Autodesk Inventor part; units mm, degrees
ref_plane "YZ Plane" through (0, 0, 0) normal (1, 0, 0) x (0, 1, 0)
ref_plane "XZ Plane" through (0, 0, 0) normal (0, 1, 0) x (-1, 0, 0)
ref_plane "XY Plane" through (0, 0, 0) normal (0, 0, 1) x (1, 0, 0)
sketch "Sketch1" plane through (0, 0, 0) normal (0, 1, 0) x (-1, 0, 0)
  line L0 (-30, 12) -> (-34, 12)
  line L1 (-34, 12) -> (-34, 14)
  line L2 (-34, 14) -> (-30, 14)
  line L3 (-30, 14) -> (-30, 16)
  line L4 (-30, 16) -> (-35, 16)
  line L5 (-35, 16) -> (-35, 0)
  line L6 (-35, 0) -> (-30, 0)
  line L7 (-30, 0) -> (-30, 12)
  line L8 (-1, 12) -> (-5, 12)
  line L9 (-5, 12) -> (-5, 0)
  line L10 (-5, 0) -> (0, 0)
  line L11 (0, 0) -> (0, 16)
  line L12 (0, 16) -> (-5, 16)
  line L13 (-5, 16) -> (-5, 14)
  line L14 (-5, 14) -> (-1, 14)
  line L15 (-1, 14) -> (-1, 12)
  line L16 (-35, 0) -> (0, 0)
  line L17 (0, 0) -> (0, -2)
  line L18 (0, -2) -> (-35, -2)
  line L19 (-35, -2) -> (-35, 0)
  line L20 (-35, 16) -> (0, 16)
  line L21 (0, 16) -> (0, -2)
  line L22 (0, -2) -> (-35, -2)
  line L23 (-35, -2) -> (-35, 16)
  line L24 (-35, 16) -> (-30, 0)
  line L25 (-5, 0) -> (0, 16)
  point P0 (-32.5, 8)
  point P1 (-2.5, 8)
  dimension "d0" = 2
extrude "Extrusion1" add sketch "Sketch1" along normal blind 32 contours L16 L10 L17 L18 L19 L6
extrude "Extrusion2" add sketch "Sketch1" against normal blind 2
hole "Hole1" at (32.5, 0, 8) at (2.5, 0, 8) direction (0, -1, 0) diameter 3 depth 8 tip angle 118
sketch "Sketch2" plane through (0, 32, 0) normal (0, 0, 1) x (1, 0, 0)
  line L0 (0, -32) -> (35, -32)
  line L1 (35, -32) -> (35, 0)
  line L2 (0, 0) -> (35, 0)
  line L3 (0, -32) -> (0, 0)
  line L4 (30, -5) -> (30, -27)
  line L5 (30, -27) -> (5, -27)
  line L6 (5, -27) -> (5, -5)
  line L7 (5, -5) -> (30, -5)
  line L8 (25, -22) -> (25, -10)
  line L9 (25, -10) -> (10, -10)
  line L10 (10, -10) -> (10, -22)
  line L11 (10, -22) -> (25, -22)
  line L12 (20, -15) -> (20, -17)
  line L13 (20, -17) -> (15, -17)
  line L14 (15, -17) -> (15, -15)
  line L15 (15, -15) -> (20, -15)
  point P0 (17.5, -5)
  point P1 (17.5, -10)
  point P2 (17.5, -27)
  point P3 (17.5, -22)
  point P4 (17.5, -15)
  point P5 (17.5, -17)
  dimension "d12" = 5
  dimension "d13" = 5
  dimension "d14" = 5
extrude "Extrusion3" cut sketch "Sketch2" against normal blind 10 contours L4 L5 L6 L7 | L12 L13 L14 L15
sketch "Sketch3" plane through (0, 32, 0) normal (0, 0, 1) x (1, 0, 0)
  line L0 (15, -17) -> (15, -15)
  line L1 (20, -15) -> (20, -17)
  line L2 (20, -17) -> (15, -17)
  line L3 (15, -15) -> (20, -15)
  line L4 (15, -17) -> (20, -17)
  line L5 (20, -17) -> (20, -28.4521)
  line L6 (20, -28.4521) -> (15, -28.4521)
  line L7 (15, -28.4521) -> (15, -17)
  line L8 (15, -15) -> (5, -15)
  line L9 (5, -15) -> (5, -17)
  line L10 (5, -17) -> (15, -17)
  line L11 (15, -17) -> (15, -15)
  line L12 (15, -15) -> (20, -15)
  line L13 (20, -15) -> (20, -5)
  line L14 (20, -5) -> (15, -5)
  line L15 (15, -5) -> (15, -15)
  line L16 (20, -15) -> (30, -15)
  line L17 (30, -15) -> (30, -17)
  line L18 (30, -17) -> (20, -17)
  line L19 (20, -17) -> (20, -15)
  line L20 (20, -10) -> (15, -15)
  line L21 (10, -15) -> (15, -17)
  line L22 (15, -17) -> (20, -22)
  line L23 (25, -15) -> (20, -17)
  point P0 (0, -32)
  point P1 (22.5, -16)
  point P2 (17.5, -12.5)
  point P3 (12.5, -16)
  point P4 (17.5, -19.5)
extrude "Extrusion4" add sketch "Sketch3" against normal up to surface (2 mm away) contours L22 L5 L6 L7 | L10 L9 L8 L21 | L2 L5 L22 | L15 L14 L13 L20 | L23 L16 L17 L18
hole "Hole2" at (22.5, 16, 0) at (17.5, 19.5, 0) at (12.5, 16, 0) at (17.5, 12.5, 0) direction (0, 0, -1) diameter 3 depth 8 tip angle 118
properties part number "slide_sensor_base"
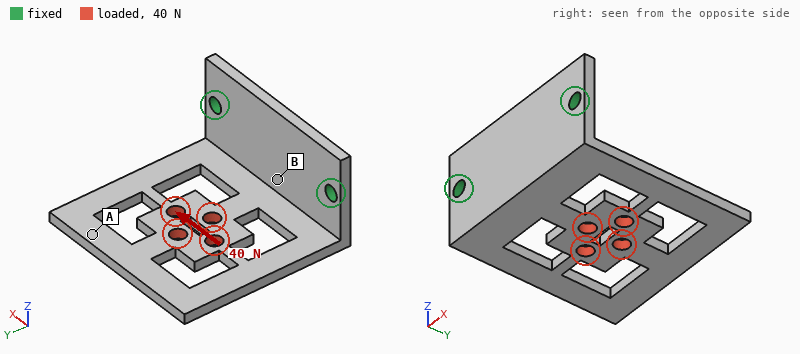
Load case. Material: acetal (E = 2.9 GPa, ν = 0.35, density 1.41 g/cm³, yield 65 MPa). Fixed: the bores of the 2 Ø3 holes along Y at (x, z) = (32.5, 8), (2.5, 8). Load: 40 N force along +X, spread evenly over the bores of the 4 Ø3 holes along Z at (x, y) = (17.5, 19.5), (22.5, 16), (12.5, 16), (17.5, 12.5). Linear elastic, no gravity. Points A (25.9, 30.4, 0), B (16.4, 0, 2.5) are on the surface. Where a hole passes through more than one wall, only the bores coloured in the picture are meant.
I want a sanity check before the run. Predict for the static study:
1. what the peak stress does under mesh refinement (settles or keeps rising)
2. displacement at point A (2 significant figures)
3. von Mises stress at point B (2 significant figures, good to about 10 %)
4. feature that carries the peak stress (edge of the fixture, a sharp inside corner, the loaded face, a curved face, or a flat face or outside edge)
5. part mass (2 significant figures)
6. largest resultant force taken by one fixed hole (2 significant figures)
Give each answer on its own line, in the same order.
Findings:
keeps rising
0.47 mm
5.7 MPa
edge of the fixture
3.9 g
33 N
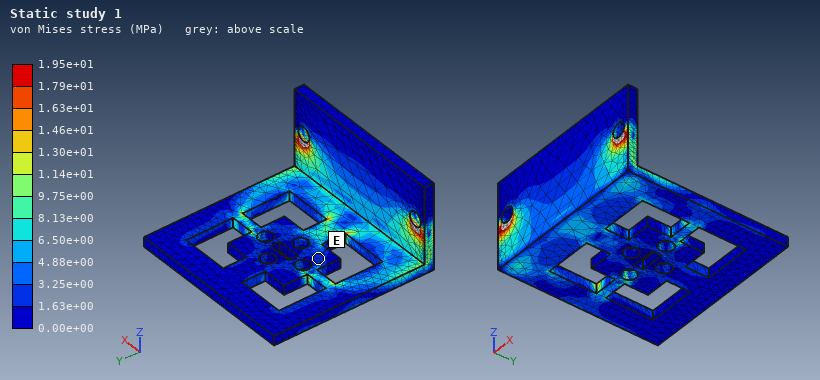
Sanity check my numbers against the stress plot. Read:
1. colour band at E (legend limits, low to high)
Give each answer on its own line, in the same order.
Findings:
1.63e+00 to 3.25e+00 MPa
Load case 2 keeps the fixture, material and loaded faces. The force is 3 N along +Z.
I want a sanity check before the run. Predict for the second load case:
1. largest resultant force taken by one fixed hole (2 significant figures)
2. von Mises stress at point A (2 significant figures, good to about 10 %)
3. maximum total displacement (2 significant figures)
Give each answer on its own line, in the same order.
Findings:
1.5 N
0.43 MPa
0.54 mm
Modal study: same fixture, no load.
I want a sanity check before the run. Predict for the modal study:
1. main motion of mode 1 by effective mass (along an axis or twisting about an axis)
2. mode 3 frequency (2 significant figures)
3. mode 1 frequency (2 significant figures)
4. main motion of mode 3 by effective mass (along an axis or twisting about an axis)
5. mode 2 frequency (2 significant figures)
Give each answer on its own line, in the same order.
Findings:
along Z
1200 Hz
290 Hz
along X
710 Hz
